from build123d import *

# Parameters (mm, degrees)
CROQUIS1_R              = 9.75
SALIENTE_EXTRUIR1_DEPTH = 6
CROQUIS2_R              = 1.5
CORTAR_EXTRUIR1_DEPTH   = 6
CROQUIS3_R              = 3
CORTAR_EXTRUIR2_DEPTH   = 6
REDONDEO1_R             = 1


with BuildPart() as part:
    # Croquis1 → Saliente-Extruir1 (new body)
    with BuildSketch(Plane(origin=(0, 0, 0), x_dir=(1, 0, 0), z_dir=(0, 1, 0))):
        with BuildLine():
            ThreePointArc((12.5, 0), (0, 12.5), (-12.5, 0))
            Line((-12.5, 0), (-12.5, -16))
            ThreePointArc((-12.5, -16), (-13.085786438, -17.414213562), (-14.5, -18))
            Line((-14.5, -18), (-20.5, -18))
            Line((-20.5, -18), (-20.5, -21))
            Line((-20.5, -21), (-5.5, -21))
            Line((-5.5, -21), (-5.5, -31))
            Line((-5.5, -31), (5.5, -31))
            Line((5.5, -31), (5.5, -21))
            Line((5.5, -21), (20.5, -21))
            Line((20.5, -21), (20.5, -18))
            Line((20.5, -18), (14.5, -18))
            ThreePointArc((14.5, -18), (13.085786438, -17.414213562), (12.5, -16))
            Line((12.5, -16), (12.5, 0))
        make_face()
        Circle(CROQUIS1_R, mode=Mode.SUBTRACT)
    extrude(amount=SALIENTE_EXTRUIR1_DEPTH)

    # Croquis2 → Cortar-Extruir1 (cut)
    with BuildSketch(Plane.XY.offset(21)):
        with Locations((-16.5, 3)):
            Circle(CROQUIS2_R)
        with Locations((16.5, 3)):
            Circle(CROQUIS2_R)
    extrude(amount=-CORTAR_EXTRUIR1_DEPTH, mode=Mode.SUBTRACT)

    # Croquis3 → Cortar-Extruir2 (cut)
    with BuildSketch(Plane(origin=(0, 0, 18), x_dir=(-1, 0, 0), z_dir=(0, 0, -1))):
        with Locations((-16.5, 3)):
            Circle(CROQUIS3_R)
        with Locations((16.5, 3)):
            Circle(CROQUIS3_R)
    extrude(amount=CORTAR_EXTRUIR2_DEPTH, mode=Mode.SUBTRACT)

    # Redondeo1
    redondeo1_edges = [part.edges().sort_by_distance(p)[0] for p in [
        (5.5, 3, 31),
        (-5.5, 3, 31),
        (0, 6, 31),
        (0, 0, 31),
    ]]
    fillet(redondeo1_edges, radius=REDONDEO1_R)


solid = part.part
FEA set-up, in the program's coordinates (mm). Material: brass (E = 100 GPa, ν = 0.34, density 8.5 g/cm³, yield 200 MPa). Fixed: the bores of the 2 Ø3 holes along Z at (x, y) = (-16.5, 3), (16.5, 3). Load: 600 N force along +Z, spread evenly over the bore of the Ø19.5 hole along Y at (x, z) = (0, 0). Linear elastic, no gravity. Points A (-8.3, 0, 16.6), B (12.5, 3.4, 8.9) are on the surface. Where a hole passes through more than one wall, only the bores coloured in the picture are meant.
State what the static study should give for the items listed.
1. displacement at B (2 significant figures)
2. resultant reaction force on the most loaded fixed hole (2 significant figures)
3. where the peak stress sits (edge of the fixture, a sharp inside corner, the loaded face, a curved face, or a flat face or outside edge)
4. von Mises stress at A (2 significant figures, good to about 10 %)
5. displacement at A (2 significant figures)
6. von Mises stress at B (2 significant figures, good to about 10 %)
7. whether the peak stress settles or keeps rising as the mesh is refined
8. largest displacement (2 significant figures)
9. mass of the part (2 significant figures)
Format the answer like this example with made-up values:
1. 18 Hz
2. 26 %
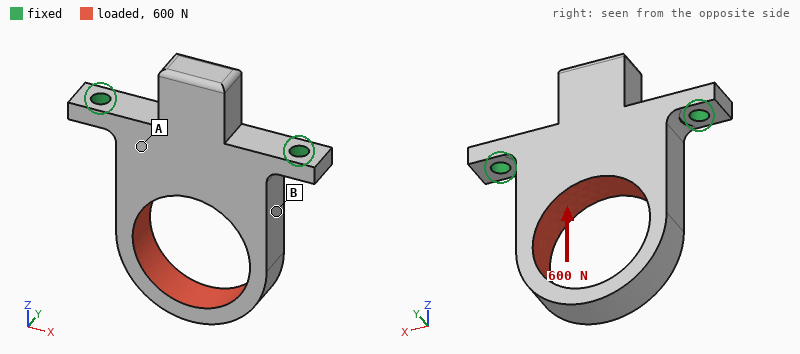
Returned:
1. 4.4 µm
2. 330 N
3. edge of the fixture
4. 6.7 MPa
5. 3.6 µm
6. 17 MPa
7. keeps rising
8. 11 µm
9. 32 g
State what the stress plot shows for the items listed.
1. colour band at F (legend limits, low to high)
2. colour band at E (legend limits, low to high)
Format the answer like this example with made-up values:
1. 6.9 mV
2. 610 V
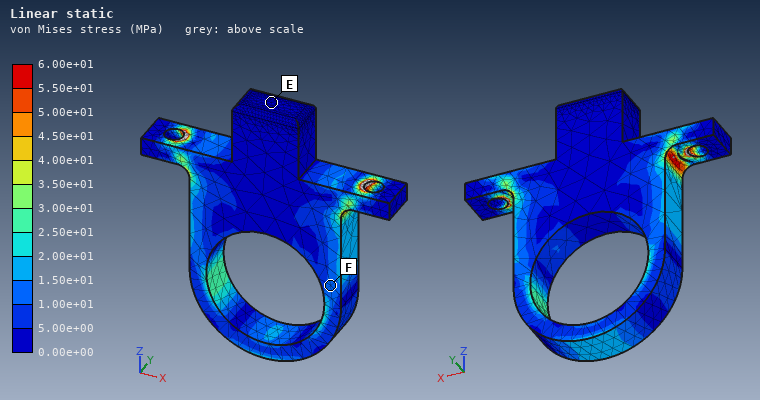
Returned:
1. 1.00e+01 to 1.50e+01 MPa
2. 0.00e+00 to 5.00e+00 MPa
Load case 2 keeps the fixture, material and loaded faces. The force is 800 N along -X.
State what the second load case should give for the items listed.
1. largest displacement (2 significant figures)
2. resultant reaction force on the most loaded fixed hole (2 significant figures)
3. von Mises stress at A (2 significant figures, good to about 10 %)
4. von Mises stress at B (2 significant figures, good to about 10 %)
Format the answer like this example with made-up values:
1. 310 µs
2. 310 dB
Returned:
1. 71 µm
2. 680 N
3. 17 MPa
4. 66 MPa
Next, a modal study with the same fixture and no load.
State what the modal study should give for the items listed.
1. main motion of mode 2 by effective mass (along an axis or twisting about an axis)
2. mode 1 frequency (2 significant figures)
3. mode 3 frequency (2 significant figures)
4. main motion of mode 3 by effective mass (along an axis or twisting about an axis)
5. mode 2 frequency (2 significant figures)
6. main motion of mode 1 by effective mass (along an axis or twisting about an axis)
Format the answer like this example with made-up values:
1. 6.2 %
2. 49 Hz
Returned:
1. along X
2. 1900 Hz
3. 7400 Hz
4. twisting about Z
5. 5900 Hz
6. along Y
